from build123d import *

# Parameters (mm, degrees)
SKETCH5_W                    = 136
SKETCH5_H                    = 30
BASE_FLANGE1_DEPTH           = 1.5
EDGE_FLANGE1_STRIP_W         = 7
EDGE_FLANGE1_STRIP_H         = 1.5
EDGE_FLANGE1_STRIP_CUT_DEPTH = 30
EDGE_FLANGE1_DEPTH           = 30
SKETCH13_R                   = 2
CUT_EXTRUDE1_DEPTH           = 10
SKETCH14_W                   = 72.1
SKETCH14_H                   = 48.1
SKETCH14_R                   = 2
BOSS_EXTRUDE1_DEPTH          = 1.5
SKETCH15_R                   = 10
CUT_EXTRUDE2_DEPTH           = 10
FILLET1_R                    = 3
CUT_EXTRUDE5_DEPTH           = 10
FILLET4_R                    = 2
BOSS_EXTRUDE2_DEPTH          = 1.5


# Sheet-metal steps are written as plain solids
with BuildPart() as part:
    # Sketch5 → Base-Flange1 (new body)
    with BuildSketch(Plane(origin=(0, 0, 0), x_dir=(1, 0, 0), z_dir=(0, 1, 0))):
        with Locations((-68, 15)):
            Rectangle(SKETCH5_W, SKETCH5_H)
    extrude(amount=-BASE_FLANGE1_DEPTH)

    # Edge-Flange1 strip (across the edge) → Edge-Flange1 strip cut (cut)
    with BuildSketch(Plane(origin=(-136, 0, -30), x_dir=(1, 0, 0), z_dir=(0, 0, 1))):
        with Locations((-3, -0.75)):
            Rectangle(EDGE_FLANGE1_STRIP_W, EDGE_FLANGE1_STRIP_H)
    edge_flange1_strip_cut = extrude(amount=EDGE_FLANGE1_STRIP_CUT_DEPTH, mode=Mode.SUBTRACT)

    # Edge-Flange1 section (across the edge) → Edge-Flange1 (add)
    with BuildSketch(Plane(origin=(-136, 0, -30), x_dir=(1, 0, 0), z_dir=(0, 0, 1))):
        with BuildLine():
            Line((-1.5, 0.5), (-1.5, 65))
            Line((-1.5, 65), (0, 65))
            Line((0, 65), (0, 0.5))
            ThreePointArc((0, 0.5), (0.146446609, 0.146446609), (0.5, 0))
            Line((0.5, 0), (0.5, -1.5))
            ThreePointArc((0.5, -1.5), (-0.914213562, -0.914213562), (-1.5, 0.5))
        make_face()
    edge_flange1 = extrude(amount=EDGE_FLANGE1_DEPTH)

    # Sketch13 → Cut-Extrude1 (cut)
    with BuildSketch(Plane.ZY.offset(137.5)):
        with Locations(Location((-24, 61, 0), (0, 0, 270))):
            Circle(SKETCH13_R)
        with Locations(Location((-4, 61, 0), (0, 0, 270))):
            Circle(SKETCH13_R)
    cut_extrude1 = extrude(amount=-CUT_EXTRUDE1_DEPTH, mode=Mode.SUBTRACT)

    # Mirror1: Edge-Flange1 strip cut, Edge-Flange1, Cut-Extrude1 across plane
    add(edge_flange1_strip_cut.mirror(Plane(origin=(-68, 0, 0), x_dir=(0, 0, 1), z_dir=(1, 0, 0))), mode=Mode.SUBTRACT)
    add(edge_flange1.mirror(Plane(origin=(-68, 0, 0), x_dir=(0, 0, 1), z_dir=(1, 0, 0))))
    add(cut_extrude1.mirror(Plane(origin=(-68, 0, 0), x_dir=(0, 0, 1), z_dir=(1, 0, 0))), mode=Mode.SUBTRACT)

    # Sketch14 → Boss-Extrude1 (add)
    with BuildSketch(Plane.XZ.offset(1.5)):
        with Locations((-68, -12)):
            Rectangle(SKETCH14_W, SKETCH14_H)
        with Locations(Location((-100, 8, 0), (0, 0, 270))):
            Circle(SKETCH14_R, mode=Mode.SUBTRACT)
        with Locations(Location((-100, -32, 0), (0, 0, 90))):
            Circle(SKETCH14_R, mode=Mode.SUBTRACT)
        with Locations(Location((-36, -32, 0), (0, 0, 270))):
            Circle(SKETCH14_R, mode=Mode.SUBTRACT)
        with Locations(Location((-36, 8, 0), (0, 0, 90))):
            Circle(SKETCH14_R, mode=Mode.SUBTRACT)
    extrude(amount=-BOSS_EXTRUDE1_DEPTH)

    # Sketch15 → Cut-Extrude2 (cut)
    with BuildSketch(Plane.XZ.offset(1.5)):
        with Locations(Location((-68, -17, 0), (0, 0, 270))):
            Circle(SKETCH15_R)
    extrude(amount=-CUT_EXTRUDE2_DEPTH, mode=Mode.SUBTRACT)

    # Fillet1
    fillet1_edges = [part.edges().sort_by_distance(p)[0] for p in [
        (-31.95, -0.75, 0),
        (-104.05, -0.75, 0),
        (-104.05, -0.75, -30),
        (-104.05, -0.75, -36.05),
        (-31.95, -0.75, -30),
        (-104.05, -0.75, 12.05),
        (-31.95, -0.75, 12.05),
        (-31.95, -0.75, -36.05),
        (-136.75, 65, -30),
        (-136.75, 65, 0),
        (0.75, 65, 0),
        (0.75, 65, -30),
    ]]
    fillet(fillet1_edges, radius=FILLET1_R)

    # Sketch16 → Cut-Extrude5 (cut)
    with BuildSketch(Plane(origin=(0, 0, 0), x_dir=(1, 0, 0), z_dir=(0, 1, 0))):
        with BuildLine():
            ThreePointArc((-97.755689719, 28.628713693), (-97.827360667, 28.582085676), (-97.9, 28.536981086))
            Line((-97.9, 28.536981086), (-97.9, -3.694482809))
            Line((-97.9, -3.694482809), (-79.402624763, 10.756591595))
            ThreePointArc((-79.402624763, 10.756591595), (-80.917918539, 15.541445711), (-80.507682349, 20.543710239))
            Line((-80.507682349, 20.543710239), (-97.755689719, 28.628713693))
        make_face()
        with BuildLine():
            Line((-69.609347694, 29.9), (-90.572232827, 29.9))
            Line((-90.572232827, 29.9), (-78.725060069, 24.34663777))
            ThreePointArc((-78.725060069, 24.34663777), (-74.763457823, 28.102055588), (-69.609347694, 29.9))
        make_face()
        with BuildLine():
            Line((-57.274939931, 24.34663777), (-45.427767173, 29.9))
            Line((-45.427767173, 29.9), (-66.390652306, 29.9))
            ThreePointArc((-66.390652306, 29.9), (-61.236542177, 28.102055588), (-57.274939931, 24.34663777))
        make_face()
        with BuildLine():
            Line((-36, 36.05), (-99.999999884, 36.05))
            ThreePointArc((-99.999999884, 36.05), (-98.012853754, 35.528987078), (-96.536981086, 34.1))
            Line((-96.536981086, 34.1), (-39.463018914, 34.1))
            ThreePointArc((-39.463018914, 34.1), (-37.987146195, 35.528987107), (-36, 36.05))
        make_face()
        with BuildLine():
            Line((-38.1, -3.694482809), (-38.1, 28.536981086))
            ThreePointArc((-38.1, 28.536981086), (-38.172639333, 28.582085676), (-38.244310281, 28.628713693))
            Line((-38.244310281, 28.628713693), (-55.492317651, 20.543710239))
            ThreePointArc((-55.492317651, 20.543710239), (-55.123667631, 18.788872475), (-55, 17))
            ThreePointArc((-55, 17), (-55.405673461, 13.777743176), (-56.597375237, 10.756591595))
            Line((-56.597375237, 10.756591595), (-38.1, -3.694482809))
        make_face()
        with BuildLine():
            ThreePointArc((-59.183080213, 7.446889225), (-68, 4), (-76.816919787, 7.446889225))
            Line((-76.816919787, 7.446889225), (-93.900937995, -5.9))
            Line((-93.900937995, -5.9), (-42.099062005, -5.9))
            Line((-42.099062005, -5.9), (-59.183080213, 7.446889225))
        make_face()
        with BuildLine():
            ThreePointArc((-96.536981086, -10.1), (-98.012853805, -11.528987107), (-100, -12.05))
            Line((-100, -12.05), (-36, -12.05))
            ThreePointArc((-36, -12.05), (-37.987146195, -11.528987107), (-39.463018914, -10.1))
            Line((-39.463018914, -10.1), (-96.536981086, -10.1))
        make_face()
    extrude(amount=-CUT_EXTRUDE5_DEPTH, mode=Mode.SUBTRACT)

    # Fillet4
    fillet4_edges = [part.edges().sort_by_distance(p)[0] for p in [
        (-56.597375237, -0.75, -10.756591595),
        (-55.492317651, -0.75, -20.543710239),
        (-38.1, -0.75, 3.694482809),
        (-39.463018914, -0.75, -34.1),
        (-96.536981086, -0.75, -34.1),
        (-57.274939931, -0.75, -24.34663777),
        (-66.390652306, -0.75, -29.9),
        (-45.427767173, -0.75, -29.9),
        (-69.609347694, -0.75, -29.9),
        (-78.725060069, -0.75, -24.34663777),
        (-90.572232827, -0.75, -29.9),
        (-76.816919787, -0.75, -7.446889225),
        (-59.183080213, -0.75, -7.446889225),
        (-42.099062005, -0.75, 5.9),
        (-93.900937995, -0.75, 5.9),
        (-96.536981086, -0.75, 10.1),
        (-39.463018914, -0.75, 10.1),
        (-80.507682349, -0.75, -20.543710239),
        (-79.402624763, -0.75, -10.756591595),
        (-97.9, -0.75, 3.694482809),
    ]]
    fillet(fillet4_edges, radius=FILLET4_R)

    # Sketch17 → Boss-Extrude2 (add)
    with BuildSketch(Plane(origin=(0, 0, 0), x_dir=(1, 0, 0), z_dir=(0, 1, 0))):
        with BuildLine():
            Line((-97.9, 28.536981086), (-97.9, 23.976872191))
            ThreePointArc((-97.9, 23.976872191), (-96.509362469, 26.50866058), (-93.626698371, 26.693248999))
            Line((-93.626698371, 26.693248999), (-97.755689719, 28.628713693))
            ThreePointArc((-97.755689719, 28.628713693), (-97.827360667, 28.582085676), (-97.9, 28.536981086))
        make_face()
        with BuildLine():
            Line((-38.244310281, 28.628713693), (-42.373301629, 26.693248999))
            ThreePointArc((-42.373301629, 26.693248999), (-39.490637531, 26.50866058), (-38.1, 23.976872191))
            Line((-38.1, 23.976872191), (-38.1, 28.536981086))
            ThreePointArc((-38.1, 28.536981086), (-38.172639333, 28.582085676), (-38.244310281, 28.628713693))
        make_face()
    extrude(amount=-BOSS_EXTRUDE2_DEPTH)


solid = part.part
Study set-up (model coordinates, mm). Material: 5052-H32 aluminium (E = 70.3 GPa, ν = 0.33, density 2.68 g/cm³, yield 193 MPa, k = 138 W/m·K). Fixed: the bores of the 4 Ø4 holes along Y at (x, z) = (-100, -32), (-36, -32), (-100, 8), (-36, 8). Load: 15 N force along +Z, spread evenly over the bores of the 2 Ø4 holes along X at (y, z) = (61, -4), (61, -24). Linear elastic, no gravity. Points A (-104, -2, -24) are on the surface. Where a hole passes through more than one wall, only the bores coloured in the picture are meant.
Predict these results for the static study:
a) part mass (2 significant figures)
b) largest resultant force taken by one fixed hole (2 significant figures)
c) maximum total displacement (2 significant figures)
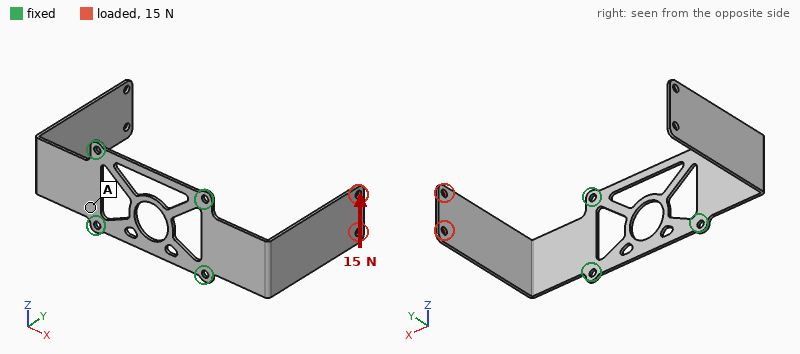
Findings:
30 g
34 N
1.9 mm
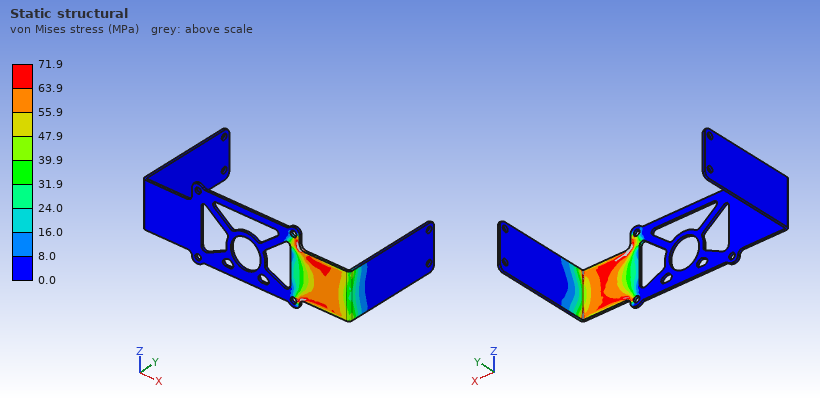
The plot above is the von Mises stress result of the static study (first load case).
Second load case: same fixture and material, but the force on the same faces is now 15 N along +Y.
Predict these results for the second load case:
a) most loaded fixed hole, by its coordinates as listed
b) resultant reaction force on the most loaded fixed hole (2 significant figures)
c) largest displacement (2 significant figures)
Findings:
(-36, -32)
8.6 N
1.6 mm
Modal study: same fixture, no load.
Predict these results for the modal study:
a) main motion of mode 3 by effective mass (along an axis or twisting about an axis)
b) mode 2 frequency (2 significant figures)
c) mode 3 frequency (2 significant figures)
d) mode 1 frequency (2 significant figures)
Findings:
along Z
140 Hz
270 Hz
140 Hz
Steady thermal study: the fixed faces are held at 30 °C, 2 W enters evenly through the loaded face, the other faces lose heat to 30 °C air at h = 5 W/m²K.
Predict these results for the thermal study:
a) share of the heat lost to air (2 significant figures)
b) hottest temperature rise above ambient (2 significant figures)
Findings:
25 %
31 K
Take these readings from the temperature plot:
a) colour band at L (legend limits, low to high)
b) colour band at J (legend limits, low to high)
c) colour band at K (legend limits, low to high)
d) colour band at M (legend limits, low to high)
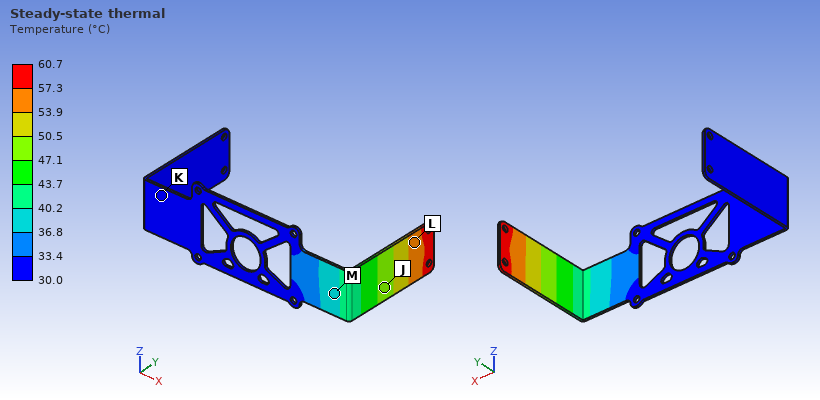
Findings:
53.9 to 57.3 °C
47.1 to 50.5 °C
30.0 to 33.4 °C
36.8 to 40.2 °C
